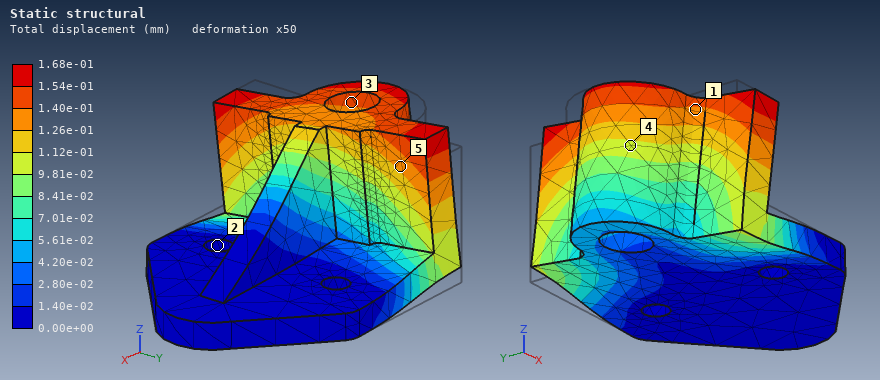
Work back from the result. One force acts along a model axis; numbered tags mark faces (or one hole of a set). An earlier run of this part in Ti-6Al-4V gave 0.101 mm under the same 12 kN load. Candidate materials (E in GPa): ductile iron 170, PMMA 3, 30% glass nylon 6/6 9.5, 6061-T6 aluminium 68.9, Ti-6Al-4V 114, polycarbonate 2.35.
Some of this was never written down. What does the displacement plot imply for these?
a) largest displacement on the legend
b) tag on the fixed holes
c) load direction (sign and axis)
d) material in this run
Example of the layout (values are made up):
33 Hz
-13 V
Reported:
1.68e-01 mm
2
-Y
6061-T6 aluminium
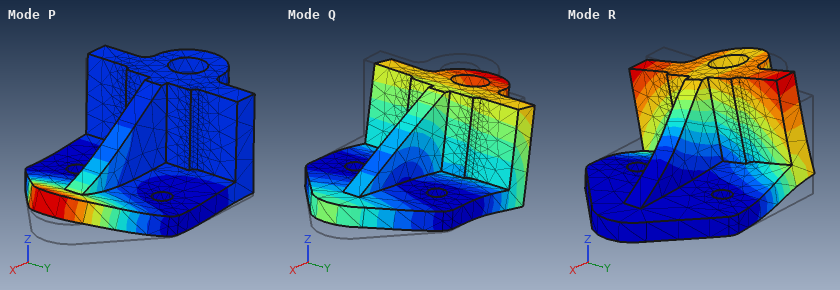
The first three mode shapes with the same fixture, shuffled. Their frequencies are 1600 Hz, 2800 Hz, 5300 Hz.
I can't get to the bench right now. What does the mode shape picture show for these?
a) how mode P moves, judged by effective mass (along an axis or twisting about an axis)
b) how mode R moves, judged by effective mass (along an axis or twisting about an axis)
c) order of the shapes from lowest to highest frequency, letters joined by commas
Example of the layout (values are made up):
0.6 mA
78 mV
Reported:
along Z
along Y
Q, R, P
